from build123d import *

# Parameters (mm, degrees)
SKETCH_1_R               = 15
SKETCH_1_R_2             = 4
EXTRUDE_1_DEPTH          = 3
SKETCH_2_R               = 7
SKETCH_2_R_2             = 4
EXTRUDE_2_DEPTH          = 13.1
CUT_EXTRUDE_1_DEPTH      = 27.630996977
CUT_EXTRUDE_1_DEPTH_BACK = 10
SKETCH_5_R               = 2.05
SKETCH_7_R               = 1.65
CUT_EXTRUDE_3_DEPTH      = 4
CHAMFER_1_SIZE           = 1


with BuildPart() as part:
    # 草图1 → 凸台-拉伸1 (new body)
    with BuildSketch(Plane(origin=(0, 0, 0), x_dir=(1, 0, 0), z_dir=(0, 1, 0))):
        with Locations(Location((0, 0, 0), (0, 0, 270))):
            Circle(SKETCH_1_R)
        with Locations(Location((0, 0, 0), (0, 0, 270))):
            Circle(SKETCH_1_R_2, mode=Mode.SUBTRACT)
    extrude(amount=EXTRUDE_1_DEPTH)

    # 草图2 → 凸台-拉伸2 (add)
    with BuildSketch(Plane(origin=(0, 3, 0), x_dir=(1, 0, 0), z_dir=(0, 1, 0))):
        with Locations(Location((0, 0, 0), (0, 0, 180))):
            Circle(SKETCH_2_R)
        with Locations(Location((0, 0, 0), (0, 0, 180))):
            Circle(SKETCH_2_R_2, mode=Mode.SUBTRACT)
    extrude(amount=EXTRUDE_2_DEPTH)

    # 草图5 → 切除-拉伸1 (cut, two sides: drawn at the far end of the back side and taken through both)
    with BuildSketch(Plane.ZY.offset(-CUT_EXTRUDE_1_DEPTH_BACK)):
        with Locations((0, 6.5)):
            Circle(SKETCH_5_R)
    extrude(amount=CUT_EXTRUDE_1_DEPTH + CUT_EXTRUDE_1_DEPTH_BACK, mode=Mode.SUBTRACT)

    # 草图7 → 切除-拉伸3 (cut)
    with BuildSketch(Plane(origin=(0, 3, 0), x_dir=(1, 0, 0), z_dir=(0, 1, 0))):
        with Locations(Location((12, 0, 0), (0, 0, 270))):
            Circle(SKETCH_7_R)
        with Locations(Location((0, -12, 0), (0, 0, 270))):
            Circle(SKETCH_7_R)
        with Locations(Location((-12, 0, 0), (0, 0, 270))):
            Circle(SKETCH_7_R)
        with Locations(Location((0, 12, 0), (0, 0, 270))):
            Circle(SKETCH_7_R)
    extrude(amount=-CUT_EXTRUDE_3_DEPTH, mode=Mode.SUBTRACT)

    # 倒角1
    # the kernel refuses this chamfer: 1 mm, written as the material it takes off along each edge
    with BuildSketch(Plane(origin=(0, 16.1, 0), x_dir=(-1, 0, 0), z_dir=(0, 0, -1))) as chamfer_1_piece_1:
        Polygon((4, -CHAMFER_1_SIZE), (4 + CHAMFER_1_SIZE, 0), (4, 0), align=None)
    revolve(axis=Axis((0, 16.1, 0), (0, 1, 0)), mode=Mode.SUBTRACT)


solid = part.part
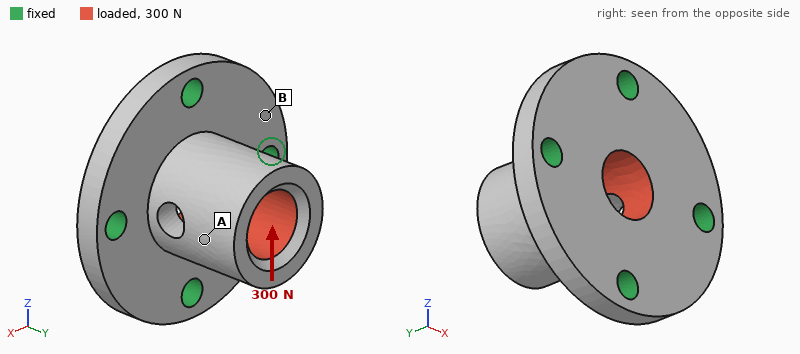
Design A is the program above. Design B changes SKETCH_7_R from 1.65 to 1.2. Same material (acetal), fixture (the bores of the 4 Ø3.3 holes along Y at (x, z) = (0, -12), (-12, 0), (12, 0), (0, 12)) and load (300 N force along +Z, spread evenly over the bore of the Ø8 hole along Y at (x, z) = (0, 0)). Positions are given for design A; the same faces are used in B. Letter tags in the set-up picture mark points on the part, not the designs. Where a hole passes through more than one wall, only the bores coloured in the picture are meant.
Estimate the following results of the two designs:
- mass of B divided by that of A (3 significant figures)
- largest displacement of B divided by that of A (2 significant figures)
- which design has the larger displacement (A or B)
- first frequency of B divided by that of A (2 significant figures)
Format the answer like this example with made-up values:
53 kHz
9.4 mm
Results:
1.02
1.1
B
0.95
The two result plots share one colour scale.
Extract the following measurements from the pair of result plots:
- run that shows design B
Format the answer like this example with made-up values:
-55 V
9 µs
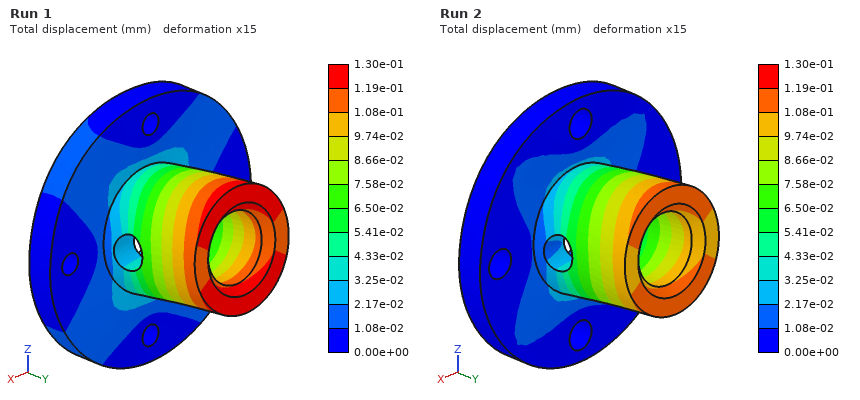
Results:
Run 1
